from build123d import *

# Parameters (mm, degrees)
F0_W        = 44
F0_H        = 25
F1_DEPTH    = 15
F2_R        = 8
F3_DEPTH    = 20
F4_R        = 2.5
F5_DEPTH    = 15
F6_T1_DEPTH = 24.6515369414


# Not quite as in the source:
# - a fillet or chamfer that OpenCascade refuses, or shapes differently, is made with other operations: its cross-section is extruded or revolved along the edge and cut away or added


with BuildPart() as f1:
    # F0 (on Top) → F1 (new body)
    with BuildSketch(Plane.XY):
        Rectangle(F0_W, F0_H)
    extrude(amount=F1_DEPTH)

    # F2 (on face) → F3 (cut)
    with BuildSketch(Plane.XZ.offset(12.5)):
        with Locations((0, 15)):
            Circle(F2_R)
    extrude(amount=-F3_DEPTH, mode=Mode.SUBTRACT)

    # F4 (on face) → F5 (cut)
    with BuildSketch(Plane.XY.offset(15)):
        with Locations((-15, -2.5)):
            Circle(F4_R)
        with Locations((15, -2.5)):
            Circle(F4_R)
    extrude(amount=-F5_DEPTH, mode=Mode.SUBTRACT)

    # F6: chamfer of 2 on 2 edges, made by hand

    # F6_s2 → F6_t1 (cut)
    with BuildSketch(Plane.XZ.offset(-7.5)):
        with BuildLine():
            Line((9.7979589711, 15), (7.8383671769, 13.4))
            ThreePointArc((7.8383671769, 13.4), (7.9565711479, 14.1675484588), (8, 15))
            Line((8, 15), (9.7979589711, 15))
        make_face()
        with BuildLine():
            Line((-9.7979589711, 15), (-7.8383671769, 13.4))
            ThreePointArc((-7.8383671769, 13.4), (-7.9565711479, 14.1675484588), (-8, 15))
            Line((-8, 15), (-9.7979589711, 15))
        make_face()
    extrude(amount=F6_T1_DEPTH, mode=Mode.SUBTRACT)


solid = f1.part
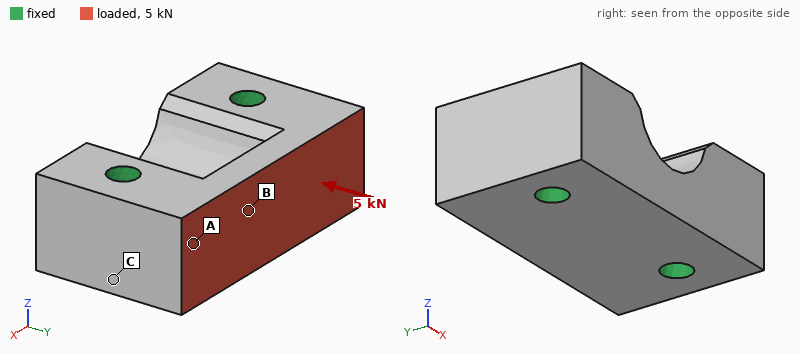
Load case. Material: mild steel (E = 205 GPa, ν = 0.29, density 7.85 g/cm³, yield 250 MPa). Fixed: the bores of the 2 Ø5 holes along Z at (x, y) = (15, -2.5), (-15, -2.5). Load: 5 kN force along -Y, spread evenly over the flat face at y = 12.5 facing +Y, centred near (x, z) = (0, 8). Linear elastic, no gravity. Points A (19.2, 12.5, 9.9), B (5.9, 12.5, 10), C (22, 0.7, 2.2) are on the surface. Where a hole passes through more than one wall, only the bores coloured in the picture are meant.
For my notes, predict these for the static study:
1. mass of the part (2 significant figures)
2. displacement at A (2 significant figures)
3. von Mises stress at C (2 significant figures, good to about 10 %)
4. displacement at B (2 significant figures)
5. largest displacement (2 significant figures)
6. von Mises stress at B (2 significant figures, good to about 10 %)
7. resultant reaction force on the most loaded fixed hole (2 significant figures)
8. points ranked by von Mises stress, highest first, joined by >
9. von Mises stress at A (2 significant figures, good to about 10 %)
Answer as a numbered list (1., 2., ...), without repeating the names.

1. 110 g
2. 0.59 µm
3. 3.8 MPa
4. 1.4 µm
5. 2.7 µm
6. 15 MPa
7. 2.5 kN
8. B > A > C
9. 8.0 MPa
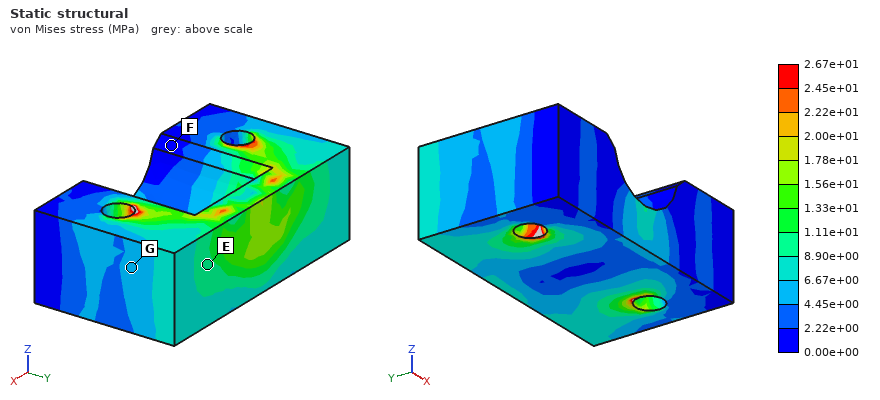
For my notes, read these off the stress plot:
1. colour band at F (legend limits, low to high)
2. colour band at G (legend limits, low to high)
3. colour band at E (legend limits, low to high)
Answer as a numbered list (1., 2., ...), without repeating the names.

1. 0.00e+00 to 2.22e+00 MPa
2. 4.45e+00 to 6.67e+00 MPa
3. 8.90e+00 to 1.11e+01 MPa
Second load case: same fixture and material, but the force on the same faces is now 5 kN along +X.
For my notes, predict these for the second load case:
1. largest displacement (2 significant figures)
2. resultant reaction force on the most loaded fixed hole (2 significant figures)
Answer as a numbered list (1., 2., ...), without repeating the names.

1. 3.9 µm
2. 3.2 kN
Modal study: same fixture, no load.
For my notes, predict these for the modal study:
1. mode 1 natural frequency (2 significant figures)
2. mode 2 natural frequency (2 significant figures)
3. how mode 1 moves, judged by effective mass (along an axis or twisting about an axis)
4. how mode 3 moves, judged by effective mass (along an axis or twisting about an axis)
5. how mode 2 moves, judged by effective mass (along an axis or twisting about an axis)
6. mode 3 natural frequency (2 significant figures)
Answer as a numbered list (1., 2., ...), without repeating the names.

1. 29 kHz
2. 36 kHz
3. along Z
4. along Y
5. along X
6. 41 kHz
